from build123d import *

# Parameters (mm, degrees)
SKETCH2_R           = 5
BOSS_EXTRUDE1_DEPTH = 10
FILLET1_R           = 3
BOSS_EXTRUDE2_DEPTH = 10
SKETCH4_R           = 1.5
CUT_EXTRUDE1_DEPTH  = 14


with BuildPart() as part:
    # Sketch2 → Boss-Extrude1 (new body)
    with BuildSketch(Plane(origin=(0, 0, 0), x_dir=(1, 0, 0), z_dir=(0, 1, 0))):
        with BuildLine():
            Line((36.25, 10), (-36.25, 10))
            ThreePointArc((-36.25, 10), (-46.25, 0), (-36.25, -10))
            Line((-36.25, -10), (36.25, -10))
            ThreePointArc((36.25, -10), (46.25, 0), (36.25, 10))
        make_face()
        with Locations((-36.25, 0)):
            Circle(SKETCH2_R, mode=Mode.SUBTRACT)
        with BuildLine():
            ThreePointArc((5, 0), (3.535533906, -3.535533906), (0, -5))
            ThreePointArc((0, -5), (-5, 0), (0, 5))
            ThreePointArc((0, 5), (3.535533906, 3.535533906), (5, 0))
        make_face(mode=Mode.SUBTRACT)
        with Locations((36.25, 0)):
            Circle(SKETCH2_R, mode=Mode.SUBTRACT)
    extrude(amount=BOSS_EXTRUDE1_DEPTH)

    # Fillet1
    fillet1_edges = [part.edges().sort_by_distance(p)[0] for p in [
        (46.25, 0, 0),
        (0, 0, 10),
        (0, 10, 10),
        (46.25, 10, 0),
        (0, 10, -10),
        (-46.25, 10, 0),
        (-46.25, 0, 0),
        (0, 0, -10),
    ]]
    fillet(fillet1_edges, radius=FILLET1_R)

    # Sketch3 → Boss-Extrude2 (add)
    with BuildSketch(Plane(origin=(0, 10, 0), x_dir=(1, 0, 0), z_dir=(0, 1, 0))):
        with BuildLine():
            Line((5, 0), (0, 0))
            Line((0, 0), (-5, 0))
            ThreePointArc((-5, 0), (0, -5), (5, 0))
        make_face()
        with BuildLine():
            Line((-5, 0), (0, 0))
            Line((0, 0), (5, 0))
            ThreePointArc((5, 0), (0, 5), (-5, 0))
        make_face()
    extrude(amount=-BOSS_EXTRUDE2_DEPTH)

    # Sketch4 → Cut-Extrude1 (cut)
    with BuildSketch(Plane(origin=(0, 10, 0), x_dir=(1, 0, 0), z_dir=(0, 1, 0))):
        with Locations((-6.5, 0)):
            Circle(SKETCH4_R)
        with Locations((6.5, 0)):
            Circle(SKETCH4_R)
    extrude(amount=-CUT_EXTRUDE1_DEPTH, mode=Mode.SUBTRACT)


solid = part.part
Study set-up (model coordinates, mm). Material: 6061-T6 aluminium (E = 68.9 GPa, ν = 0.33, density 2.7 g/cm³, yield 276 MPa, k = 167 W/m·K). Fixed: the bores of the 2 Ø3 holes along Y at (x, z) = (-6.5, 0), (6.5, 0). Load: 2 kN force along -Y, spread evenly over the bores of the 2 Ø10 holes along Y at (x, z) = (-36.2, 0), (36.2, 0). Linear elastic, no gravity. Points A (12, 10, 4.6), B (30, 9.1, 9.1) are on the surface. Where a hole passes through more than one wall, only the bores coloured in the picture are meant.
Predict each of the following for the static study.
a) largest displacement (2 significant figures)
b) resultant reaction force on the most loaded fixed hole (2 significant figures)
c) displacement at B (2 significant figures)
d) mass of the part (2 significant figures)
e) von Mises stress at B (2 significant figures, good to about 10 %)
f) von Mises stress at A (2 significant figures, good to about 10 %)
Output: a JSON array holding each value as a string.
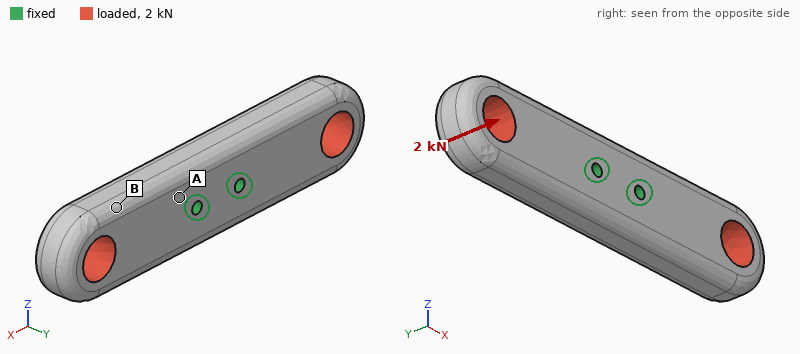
["0.16 mm", "1.0 kN", "0.074 mm", "41 g", "26 MPa", "72 MPa"]
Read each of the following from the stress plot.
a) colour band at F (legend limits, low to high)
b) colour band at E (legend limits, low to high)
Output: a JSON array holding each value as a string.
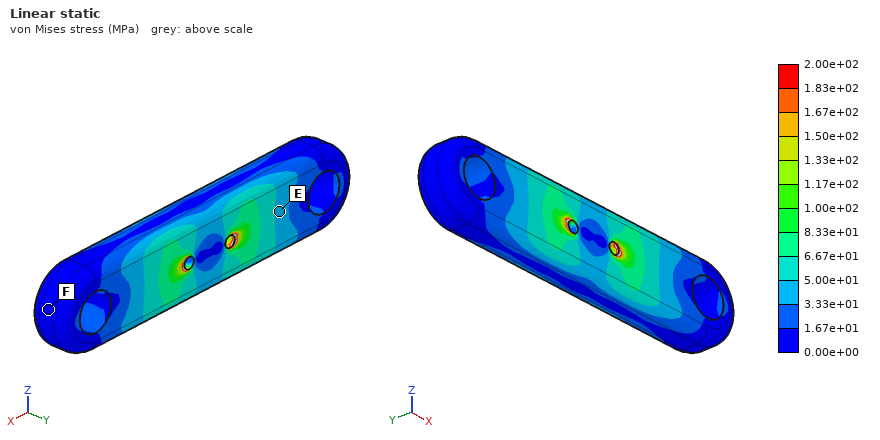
["0.00e+00 to 1.67e+01 MPa", "3.33e+01 to 5.00e+01 MPa"]
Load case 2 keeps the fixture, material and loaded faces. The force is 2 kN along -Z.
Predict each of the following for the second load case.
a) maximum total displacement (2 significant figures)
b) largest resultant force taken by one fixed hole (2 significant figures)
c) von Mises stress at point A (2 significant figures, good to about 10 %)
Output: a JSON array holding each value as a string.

["61 µm", "1.0 kN", "21 MPa"]
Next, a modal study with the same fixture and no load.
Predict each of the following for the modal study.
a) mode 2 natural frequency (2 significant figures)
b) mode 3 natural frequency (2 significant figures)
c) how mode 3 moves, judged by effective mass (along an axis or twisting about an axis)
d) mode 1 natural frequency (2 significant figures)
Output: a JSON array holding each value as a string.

["5700 Hz", "7000 Hz", "twisting about Y", "5600 Hz"]
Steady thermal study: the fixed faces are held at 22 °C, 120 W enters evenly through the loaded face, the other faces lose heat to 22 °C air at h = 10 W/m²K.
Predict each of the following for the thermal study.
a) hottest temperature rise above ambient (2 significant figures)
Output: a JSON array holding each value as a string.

["73 K"]
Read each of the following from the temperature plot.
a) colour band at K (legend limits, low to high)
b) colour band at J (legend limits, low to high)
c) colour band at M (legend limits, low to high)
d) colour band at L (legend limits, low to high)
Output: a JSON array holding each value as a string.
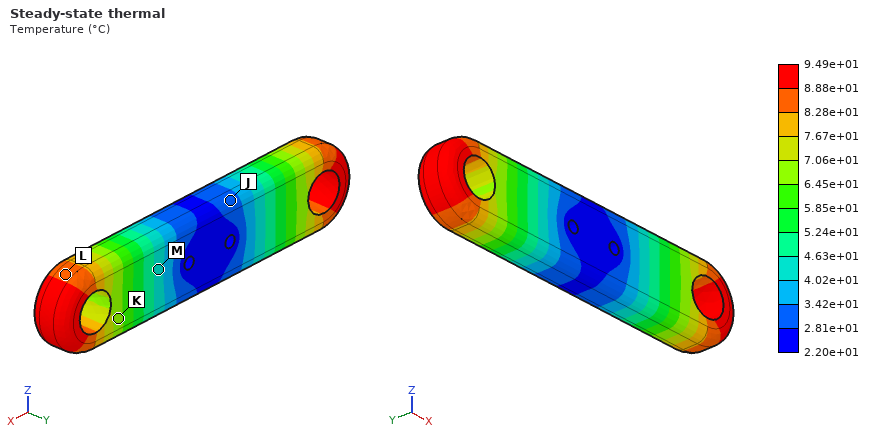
["6.45e+01 to 7.06e+01 °C", "2.81e+01 to 3.42e+01 °C", "4.02e+01 to 4.63e+01 °C", "8.28e+01 to 8.88e+01 °C"]
